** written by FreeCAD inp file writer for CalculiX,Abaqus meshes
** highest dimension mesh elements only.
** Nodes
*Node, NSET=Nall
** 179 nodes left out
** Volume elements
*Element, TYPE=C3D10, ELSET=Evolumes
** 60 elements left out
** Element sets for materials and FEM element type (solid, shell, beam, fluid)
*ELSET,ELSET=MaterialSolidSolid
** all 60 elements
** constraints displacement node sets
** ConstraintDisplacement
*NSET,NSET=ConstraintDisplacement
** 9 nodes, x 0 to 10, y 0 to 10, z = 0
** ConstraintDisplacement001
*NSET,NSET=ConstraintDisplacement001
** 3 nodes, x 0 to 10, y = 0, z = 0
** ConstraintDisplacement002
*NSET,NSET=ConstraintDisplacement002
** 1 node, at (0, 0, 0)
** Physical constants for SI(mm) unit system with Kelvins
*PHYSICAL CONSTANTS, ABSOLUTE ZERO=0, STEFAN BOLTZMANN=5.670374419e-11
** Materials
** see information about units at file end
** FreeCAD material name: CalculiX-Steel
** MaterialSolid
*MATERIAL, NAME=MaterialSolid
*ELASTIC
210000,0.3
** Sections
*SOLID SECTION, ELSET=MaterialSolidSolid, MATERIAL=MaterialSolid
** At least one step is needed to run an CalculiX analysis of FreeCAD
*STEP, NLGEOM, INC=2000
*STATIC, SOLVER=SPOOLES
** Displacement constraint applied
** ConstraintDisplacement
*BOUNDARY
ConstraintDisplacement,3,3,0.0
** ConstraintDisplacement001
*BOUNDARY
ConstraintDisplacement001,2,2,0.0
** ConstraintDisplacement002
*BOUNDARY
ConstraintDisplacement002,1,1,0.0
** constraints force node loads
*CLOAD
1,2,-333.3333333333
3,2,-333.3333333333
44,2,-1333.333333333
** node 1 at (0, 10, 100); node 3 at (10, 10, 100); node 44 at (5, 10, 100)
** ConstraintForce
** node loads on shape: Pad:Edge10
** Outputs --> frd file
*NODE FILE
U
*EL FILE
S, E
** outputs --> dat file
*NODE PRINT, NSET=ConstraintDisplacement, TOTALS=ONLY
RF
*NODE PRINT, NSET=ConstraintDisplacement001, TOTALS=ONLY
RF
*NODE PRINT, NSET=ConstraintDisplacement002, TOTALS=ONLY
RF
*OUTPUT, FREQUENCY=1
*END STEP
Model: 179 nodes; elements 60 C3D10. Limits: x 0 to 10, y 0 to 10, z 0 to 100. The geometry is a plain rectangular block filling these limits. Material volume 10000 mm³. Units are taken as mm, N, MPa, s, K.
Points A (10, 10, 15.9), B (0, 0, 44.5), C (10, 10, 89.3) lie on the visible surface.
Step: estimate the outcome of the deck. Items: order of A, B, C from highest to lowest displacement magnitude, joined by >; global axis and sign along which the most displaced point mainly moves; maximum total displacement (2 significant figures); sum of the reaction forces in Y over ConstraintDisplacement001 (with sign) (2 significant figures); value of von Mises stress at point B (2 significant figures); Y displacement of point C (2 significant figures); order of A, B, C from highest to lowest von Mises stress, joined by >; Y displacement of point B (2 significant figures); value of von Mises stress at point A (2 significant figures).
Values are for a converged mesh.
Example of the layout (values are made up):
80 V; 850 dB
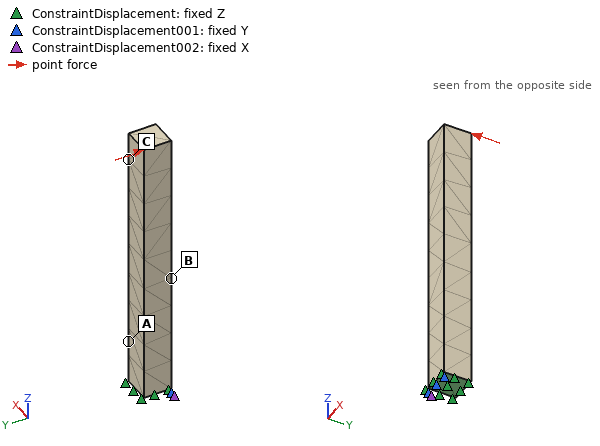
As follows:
C > B > A; -Y; 3.9 mm; 2000 N; 660 MPa; -3.2 mm; A > B > C; -0.97 mm; 1000 MPa
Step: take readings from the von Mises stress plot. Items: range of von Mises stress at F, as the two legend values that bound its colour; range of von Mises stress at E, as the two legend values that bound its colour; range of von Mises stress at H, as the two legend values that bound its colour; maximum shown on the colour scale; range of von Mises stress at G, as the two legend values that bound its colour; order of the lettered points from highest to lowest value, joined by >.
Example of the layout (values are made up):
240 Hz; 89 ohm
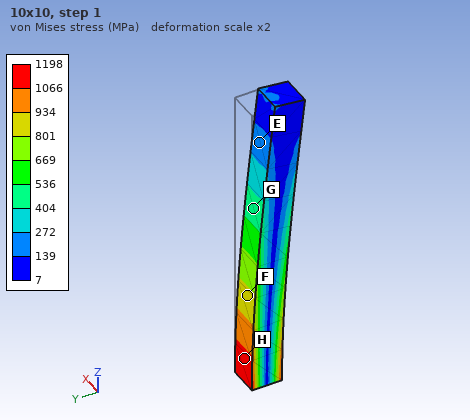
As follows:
801 to 934 MPa; 139 to 272 MPa; 1066 to 1198 MPa; 1198 MPa; 404 to 536 MPa; H > F > G > E
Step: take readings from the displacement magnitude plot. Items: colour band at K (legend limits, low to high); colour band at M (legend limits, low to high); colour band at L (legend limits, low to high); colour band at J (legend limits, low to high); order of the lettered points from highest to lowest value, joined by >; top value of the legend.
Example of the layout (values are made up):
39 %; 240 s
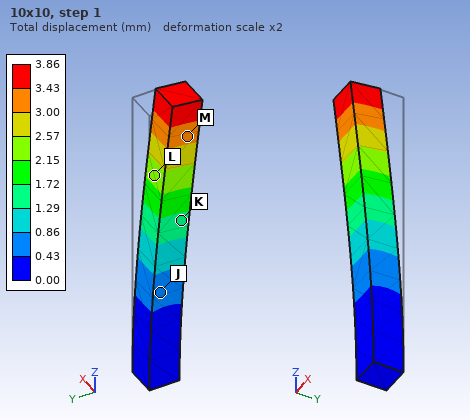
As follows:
1.29 to 1.72 mm; 3.00 to 3.43 mm; 2.15 to 2.57 mm; 0.43 to 0.86 mm; M > L > K > J; 3.86 mm
